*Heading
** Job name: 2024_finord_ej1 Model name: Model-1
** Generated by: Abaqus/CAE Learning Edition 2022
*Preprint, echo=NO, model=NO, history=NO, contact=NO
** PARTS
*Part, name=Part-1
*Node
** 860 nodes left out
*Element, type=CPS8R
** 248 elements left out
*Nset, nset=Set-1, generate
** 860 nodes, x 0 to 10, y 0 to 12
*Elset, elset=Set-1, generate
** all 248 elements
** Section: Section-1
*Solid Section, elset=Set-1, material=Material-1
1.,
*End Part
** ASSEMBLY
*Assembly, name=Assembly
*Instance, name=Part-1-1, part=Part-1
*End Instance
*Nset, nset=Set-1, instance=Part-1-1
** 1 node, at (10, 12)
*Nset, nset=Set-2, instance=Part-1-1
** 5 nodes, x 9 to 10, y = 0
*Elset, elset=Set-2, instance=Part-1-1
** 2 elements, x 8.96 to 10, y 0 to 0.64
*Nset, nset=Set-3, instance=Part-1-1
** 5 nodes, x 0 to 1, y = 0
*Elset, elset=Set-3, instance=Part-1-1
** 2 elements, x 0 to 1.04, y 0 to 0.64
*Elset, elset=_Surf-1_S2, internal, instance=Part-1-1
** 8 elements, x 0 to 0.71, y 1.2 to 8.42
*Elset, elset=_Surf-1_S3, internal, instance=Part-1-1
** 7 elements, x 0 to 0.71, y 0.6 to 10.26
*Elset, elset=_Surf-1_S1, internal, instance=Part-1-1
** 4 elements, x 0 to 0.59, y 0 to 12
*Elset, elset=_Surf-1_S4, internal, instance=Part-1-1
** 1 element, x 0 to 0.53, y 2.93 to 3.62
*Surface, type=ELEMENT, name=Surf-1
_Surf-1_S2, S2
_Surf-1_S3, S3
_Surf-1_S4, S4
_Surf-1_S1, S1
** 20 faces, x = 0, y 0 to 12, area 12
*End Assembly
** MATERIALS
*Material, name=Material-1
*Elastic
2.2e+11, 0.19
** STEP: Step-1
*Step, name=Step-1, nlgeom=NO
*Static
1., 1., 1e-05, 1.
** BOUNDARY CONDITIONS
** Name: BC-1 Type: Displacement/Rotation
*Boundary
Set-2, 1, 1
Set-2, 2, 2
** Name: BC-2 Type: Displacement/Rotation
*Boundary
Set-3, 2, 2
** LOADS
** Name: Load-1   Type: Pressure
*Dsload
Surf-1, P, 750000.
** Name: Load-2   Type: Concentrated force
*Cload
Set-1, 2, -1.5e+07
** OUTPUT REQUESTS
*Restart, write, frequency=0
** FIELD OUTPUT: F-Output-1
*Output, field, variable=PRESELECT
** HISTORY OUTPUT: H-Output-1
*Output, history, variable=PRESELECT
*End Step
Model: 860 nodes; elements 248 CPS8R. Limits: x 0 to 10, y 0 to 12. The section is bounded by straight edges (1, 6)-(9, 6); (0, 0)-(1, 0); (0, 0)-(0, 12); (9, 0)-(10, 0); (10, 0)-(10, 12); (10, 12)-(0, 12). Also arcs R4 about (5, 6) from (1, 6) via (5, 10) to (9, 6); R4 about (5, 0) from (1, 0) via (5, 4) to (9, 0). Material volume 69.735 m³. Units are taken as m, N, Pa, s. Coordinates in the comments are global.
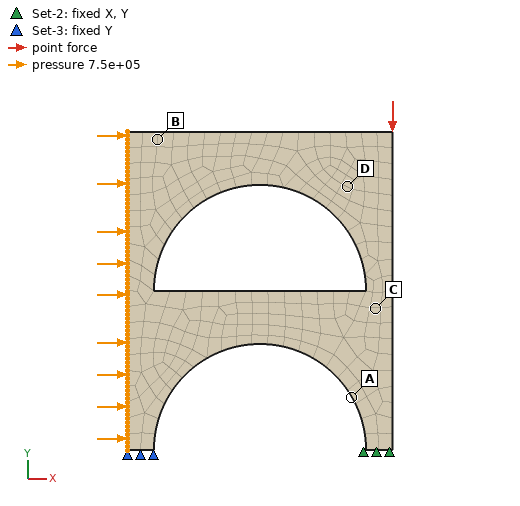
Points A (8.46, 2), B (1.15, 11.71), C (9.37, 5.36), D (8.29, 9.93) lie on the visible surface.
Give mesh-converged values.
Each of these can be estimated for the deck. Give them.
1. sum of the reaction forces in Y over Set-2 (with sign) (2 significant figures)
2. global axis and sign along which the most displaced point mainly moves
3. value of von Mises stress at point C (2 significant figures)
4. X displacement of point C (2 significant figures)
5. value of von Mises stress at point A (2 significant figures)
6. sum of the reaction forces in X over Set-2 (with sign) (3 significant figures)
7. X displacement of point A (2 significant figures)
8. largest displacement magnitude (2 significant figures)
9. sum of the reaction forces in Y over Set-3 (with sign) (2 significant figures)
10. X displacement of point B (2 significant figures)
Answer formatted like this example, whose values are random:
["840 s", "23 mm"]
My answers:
["2.1e+07 N", "+X", "1.5e+07 Pa", "0.0017 m", "2.6e+07 Pa", "-9.00e+06 N", "7.3e-04 m", "0.0031 m", "-6.0e+06 N", "0.0025 m"]
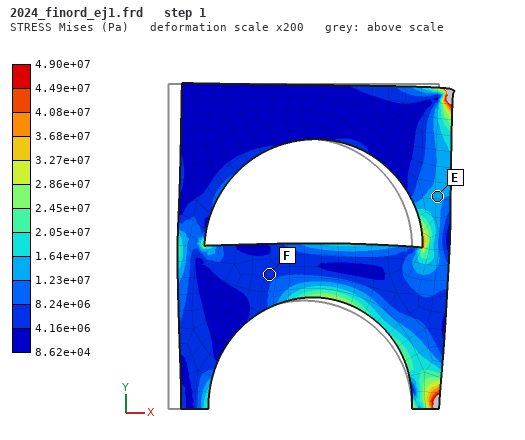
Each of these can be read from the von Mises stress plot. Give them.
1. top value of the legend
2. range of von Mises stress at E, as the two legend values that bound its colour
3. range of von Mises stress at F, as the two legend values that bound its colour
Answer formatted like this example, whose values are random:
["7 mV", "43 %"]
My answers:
["4.90e+07 Pa", "1.23e+07 to 1.64e+07 Pa", "4.16e+06 to 8.24e+06 Pa"]
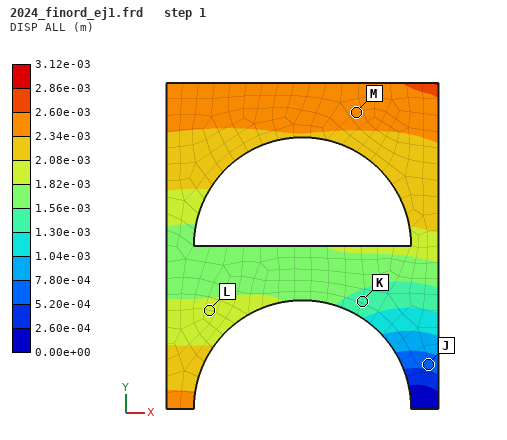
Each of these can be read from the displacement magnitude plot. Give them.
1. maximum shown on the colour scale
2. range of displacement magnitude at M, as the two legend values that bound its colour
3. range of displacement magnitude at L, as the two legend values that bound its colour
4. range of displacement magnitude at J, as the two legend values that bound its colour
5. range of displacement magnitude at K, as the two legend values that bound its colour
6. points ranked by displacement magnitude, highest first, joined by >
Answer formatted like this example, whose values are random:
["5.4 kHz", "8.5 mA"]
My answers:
["3.12e-03 m", "2.34e-03 to 2.60e-03 m", "1.82e-03 to 2.08e-03 m", "5.20e-04 to 7.80e-04 m", "1.30e-03 to 1.56e-03 m", "M > L > K > J"]
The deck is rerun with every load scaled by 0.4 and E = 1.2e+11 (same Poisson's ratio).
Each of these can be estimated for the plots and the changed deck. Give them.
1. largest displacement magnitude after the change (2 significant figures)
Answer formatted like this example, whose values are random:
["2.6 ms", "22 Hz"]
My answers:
["0.0023 m"]
